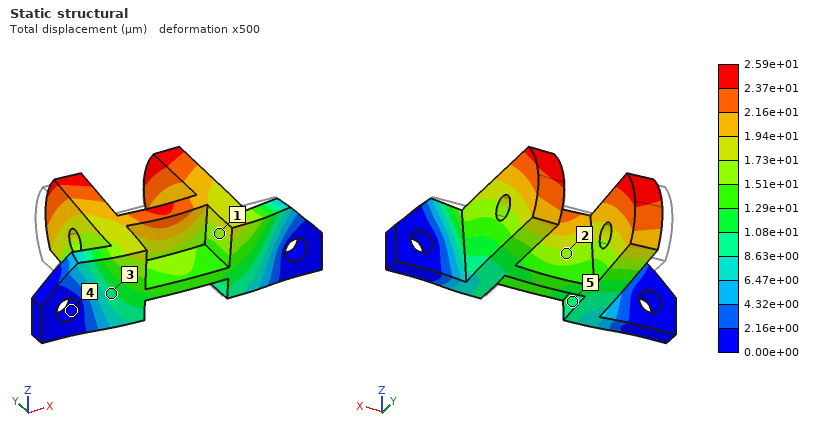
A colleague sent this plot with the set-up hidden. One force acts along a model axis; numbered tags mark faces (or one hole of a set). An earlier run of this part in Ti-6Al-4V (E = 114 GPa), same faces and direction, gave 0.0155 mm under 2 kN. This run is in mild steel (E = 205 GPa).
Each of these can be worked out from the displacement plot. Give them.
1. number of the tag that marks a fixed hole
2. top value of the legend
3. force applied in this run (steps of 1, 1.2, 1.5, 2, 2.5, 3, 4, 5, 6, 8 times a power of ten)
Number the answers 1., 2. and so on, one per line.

1. 4
2. 2.59e+01 µm
3. 6 kN
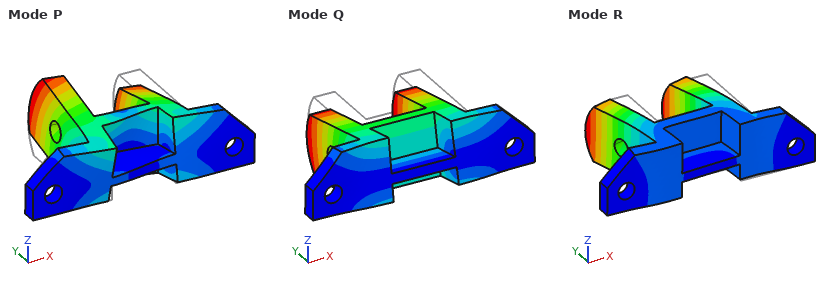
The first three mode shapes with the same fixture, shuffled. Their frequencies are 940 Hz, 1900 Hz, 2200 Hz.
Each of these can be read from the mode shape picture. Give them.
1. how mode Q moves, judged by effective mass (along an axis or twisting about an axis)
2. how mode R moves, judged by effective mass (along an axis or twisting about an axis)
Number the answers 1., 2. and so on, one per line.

1. along Z
2. along X
